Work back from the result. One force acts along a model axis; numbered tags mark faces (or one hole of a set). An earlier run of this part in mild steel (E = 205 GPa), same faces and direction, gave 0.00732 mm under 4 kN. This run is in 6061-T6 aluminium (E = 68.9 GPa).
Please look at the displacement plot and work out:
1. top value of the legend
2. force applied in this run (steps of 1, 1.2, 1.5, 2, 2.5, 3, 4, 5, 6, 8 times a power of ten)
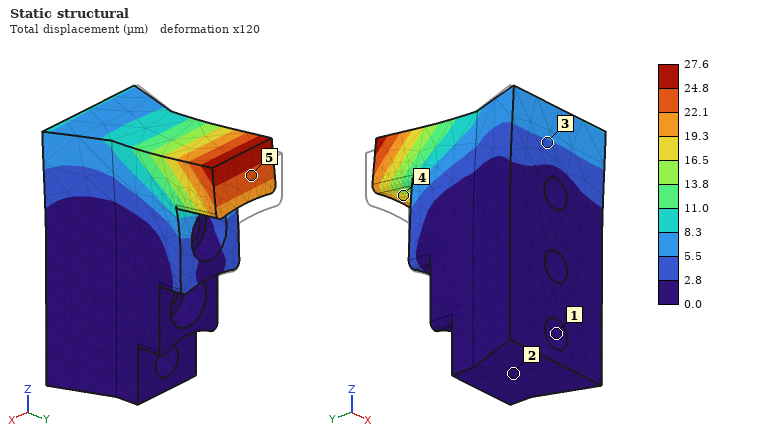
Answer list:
27.6 µm
5 kN
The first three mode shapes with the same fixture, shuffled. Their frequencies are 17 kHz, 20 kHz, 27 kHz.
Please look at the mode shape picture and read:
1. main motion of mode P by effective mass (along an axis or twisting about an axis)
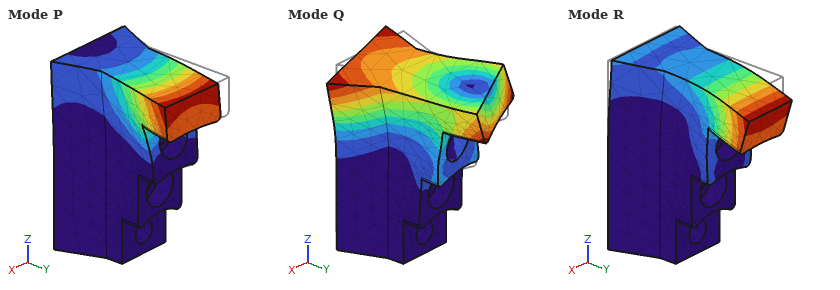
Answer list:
along X
